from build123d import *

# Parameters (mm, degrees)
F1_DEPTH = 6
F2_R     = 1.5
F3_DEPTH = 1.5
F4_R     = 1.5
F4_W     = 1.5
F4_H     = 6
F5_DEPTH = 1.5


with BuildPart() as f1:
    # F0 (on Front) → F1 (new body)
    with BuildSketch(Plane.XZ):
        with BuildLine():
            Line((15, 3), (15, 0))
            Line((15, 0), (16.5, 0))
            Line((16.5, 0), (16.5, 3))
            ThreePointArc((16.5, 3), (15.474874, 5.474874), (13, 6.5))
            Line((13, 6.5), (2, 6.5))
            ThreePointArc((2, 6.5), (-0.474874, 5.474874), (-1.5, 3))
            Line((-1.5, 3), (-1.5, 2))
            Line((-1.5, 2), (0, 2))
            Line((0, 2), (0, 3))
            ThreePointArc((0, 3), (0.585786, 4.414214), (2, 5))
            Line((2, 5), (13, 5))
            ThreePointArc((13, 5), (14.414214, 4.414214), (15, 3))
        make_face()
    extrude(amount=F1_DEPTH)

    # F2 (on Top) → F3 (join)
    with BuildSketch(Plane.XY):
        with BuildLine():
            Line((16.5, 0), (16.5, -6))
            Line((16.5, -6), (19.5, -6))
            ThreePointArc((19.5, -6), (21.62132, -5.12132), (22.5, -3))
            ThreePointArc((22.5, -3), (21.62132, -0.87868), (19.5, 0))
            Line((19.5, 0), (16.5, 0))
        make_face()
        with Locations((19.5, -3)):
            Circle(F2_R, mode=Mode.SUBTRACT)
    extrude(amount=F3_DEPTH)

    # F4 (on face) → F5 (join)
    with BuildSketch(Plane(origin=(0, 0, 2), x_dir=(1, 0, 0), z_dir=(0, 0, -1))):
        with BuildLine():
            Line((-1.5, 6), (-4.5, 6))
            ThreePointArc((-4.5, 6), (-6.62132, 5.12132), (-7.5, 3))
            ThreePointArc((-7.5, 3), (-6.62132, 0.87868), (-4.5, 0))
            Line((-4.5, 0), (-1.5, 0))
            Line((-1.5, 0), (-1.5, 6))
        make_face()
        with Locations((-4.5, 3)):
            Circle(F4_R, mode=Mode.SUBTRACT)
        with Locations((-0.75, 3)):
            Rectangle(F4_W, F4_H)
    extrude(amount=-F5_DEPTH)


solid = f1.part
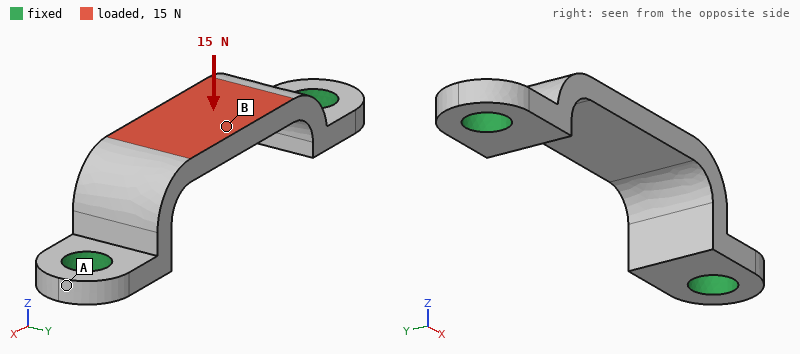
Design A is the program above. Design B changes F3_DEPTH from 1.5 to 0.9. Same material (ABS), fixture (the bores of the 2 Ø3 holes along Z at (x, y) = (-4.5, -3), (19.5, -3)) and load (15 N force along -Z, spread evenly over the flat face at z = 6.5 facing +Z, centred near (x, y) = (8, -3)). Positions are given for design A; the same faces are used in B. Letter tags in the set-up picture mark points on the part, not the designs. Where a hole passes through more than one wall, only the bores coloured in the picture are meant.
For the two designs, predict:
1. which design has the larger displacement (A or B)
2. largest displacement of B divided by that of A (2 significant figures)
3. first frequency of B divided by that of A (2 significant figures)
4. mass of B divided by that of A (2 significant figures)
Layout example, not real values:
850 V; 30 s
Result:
B; 1.1; 0.73; 0.95
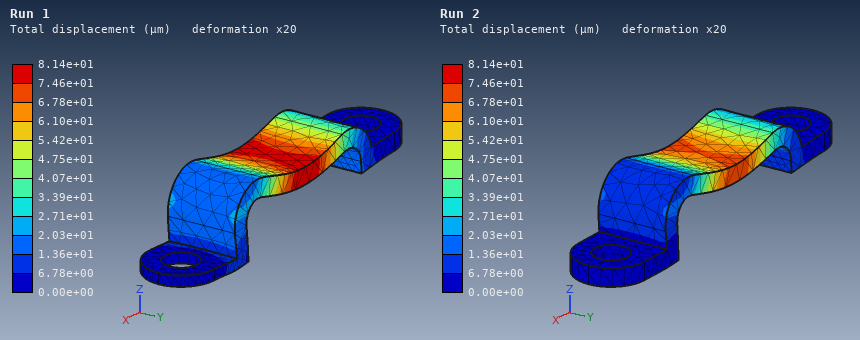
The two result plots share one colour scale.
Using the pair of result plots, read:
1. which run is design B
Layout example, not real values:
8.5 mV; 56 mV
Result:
Run 1
